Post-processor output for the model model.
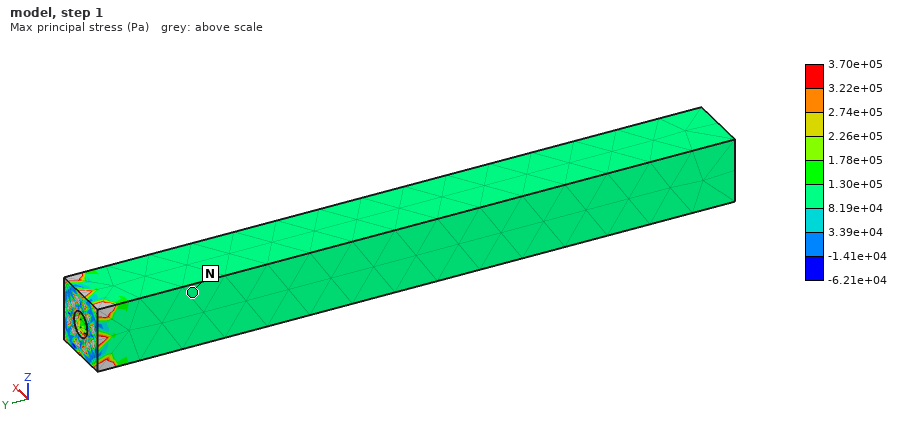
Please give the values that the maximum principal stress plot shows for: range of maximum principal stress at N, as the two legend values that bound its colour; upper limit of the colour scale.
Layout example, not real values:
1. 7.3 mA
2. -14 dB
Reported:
1. 8.19e+04 to 1.30e+05 Pa
2. 3.70e+05 Pa
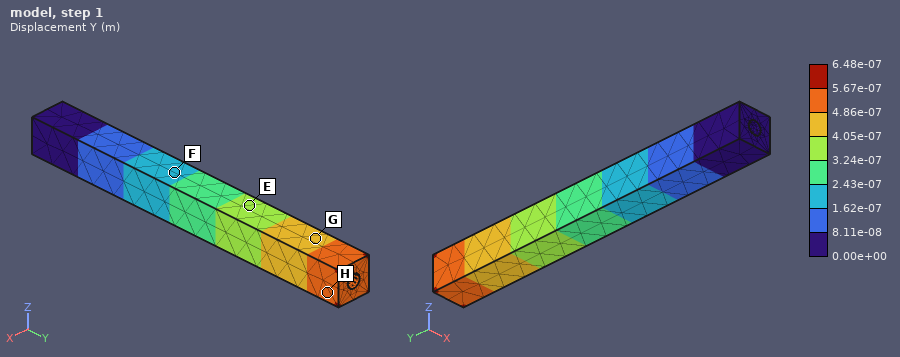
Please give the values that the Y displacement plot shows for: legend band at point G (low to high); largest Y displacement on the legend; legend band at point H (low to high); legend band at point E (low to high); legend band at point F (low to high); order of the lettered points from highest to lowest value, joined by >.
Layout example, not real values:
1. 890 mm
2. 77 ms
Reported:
1. 4.05e-07 to 4.86e-07 m
2. 6.48e-07 m
3. 4.86e-07 to 5.67e-07 m
4. 3.24e-07 to 4.05e-07 m
5. 1.62e-07 to 2.43e-07 m
6. H > G > E > F
